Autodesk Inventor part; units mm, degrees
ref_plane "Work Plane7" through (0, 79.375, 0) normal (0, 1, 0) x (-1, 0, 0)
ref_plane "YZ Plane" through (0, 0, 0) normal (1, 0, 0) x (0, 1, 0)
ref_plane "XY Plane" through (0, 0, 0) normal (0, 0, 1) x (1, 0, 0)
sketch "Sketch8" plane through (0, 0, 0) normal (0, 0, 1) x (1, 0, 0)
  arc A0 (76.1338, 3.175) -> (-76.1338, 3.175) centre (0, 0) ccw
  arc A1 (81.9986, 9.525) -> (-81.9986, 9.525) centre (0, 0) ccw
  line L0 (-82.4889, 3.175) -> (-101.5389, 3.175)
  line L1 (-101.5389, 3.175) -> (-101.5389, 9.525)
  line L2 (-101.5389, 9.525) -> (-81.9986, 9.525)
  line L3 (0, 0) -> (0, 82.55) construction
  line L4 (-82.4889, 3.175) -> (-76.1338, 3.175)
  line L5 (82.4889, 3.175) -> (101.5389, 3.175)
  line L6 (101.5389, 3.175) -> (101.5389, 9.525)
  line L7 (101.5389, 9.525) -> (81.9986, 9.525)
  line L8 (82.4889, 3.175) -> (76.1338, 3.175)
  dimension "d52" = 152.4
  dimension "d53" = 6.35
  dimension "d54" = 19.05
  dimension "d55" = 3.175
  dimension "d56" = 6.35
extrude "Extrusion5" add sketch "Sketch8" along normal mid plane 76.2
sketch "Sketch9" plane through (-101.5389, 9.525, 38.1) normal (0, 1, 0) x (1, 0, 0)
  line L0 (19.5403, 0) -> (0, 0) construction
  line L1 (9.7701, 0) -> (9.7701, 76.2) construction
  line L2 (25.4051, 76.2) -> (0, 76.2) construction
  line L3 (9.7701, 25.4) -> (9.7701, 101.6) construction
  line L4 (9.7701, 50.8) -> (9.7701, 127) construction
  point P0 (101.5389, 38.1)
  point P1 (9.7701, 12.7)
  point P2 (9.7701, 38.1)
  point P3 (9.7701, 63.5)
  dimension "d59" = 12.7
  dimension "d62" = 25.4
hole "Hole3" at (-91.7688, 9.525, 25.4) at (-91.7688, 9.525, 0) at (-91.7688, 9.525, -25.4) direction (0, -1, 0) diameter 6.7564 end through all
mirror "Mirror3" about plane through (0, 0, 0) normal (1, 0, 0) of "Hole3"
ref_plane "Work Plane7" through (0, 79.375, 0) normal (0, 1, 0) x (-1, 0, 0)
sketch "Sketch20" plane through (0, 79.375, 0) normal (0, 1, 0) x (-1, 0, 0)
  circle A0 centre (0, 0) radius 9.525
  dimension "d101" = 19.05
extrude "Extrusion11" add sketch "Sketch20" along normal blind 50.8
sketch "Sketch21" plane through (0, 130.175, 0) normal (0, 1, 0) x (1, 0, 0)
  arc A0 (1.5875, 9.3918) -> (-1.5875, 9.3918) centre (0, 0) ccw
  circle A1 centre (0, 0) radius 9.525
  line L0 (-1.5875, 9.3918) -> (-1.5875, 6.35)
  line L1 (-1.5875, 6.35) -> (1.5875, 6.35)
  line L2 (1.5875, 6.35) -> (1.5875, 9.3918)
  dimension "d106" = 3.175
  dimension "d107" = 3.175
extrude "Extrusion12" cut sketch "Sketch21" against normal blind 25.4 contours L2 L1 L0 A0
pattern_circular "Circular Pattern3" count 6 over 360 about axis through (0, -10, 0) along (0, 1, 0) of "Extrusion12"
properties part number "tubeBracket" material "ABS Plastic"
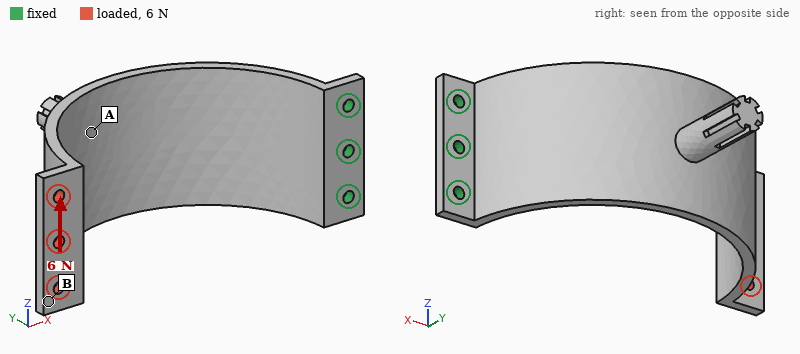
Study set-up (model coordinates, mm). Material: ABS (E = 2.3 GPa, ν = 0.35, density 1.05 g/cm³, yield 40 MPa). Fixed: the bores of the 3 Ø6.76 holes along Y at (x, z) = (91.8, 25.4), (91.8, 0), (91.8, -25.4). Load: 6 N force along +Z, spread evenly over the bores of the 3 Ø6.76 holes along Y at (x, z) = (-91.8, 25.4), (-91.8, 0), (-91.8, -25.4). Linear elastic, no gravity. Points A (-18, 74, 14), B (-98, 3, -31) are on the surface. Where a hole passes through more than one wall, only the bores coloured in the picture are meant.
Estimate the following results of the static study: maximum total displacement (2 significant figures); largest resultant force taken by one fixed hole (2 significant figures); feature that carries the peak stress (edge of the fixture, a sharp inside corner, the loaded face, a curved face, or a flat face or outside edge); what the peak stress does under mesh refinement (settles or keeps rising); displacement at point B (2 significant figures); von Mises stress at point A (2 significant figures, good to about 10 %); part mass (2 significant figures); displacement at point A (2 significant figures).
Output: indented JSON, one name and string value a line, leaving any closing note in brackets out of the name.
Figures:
{
  "maximum total displacement": "2.3 mm",
  "largest resultant force taken by one fixed hole": "20 N",
  "feature that carries the peak stress": "edge of the fixture",
  "what the peak stress does under mesh refinement": "keeps rising",
  "displacement at point B": "2.3 mm",
  "von Mises stress at point A": "0.52 MPa",
  "part mass": "150 g",
  "displacement at point A": "0.63 mm"
}
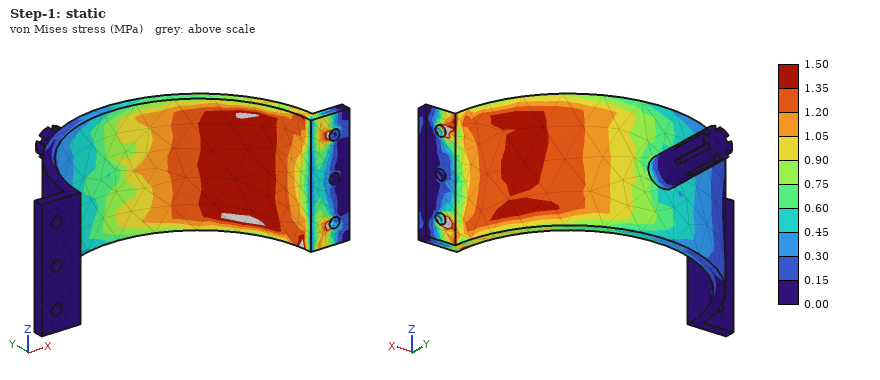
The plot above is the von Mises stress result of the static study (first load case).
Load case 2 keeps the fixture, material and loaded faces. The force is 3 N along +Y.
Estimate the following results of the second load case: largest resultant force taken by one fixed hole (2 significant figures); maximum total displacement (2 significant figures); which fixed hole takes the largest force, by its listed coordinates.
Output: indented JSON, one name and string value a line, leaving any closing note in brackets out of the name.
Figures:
{
  "largest resultant force taken by one fixed hole": "4.8 N",
  "maximum total displacement": "2.5 mm",
  "which fixed hole takes the largest force, by its listed coordinates": "(91.8, 0)"
}
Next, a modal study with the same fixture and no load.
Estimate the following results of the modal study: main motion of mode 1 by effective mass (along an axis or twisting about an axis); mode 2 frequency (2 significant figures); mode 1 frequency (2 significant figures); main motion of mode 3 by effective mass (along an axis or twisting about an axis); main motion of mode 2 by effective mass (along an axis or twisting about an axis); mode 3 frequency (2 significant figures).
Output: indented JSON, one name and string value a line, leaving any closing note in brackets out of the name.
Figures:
{
  "main motion of mode 1 by effective mass": "along Y",
  "mode 2 frequency": "46 Hz",
  "mode 1 frequency": "26 Hz",
  "main motion of mode 3 by effective mass": "along X",
  "main motion of mode 2 by effective mass": "along Z",
  "mode 3 frequency": "84 Hz"
}
